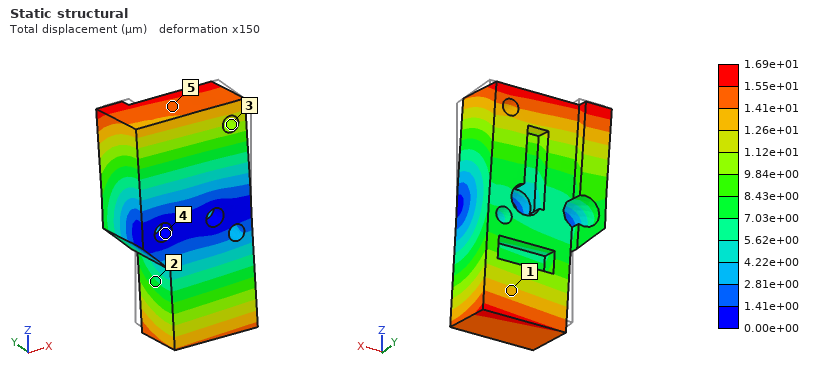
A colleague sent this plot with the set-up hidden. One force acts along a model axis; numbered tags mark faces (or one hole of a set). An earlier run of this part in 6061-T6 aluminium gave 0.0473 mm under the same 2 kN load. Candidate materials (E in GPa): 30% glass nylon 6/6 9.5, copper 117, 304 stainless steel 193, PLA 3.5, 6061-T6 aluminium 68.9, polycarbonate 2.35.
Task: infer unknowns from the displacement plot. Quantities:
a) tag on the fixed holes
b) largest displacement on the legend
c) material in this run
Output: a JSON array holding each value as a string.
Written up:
["4", "1.69e+01 µm", "304 stainless steel"]
